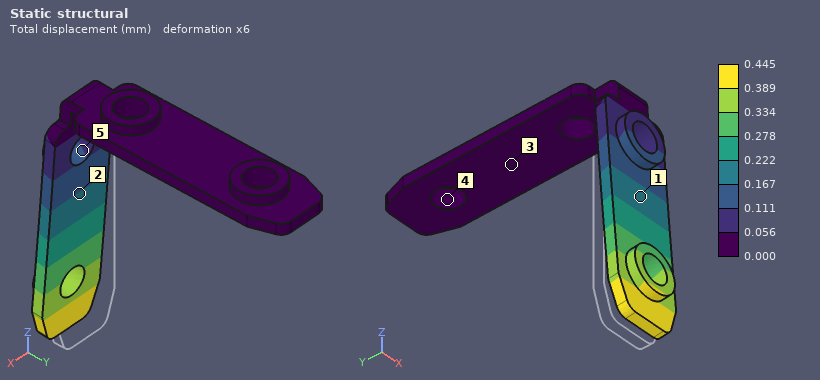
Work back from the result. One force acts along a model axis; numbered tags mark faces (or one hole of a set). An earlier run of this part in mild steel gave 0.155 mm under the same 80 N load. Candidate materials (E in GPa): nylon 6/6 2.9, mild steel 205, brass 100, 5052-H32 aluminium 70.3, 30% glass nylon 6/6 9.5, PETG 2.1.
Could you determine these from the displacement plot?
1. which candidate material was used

5052-H32 aluminium
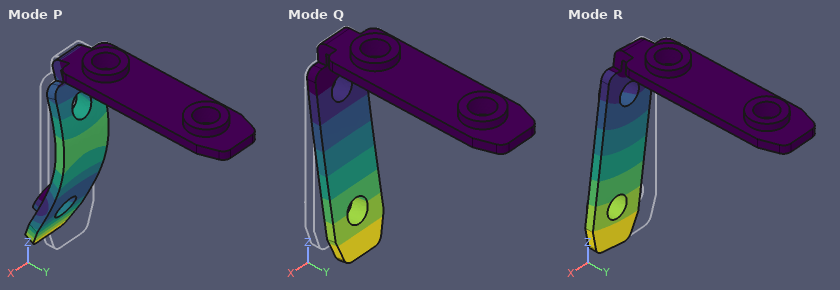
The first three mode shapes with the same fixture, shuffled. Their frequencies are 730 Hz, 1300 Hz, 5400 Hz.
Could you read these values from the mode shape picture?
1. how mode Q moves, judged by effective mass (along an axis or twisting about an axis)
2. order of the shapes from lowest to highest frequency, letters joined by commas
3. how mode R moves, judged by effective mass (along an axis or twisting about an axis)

along Y
Q, R, P
along X
